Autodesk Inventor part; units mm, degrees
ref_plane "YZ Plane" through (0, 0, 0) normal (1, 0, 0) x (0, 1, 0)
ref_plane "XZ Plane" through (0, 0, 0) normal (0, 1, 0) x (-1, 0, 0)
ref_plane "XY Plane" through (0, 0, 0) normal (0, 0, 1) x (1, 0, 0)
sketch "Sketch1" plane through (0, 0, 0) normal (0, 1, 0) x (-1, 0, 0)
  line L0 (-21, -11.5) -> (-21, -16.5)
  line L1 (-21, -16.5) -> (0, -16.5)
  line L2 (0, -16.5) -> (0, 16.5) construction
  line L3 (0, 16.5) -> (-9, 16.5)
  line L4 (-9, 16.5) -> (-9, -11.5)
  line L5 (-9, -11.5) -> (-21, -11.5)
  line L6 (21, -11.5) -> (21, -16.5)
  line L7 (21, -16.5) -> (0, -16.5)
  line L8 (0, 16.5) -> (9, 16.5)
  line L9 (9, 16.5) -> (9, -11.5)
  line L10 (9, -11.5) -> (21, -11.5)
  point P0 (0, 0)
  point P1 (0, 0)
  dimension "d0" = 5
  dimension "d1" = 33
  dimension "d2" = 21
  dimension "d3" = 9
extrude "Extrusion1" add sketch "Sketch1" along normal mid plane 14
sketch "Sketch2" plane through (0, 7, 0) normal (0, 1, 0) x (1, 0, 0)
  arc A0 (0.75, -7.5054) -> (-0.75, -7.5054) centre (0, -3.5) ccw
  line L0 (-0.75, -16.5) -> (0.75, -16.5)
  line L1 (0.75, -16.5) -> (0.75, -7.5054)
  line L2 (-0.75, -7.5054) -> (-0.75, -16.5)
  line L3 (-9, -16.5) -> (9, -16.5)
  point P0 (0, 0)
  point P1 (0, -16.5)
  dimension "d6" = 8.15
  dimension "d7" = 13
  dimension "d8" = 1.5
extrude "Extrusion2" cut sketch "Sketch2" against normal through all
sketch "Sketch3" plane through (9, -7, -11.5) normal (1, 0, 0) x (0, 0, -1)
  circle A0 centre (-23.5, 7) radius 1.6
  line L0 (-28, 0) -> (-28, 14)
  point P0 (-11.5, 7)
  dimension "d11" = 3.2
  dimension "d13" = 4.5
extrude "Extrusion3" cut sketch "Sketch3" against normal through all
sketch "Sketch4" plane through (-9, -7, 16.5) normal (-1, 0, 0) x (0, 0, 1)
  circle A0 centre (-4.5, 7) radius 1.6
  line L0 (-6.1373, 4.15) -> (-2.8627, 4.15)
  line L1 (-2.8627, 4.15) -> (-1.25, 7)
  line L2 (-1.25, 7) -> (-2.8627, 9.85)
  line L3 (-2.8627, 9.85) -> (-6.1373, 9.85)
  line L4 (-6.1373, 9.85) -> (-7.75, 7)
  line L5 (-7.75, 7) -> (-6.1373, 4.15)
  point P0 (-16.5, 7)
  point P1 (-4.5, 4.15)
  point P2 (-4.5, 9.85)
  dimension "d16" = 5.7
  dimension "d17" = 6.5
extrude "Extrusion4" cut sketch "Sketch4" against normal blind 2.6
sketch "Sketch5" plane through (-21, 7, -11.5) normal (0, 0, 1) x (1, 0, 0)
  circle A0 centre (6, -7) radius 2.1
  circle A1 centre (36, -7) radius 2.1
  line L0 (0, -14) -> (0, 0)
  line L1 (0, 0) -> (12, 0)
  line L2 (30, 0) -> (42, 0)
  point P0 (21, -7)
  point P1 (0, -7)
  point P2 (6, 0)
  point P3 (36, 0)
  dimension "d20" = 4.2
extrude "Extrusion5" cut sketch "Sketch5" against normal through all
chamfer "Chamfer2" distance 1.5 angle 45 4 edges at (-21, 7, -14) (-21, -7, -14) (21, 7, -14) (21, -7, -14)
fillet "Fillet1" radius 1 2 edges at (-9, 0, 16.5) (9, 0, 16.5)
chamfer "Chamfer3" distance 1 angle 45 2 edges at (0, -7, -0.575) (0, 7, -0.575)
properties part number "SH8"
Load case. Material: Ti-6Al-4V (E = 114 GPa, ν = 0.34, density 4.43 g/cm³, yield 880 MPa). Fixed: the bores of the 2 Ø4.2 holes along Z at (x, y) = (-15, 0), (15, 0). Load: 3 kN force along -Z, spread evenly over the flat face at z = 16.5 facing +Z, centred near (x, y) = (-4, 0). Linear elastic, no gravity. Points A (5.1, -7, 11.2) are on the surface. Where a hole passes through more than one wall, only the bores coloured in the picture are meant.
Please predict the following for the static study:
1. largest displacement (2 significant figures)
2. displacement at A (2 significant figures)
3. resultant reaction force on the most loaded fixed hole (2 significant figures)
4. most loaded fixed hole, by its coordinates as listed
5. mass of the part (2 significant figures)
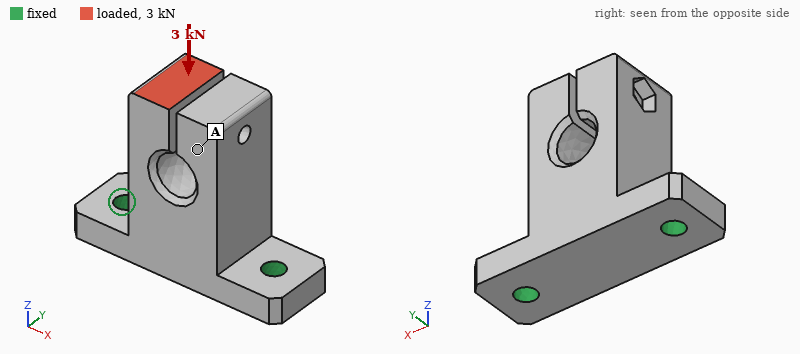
42 µm
11 µm
2.1 kN
(-15, 0)
39 g
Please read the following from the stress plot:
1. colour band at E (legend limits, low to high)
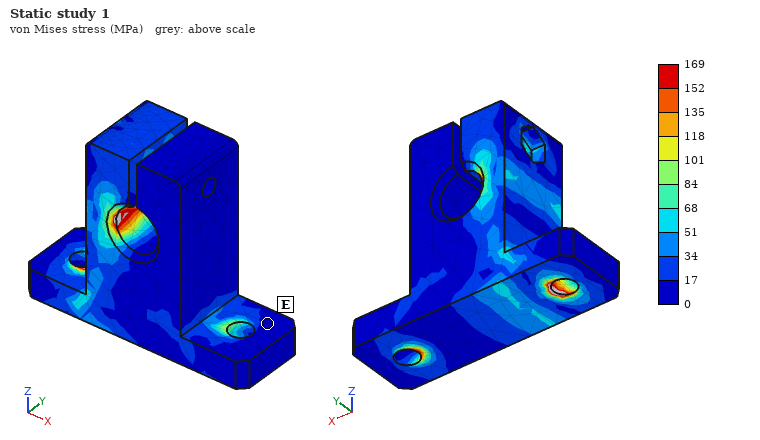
0 to 17 MPa
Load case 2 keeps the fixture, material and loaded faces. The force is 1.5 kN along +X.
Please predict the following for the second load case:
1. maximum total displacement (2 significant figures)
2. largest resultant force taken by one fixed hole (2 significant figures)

0.21 mm
2.2 kN
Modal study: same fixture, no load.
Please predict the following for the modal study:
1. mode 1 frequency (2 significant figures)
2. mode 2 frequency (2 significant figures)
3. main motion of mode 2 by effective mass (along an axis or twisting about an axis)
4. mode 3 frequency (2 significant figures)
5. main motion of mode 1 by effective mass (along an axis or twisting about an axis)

4200 Hz
7600 Hz
along X
9700 Hz
along Y
